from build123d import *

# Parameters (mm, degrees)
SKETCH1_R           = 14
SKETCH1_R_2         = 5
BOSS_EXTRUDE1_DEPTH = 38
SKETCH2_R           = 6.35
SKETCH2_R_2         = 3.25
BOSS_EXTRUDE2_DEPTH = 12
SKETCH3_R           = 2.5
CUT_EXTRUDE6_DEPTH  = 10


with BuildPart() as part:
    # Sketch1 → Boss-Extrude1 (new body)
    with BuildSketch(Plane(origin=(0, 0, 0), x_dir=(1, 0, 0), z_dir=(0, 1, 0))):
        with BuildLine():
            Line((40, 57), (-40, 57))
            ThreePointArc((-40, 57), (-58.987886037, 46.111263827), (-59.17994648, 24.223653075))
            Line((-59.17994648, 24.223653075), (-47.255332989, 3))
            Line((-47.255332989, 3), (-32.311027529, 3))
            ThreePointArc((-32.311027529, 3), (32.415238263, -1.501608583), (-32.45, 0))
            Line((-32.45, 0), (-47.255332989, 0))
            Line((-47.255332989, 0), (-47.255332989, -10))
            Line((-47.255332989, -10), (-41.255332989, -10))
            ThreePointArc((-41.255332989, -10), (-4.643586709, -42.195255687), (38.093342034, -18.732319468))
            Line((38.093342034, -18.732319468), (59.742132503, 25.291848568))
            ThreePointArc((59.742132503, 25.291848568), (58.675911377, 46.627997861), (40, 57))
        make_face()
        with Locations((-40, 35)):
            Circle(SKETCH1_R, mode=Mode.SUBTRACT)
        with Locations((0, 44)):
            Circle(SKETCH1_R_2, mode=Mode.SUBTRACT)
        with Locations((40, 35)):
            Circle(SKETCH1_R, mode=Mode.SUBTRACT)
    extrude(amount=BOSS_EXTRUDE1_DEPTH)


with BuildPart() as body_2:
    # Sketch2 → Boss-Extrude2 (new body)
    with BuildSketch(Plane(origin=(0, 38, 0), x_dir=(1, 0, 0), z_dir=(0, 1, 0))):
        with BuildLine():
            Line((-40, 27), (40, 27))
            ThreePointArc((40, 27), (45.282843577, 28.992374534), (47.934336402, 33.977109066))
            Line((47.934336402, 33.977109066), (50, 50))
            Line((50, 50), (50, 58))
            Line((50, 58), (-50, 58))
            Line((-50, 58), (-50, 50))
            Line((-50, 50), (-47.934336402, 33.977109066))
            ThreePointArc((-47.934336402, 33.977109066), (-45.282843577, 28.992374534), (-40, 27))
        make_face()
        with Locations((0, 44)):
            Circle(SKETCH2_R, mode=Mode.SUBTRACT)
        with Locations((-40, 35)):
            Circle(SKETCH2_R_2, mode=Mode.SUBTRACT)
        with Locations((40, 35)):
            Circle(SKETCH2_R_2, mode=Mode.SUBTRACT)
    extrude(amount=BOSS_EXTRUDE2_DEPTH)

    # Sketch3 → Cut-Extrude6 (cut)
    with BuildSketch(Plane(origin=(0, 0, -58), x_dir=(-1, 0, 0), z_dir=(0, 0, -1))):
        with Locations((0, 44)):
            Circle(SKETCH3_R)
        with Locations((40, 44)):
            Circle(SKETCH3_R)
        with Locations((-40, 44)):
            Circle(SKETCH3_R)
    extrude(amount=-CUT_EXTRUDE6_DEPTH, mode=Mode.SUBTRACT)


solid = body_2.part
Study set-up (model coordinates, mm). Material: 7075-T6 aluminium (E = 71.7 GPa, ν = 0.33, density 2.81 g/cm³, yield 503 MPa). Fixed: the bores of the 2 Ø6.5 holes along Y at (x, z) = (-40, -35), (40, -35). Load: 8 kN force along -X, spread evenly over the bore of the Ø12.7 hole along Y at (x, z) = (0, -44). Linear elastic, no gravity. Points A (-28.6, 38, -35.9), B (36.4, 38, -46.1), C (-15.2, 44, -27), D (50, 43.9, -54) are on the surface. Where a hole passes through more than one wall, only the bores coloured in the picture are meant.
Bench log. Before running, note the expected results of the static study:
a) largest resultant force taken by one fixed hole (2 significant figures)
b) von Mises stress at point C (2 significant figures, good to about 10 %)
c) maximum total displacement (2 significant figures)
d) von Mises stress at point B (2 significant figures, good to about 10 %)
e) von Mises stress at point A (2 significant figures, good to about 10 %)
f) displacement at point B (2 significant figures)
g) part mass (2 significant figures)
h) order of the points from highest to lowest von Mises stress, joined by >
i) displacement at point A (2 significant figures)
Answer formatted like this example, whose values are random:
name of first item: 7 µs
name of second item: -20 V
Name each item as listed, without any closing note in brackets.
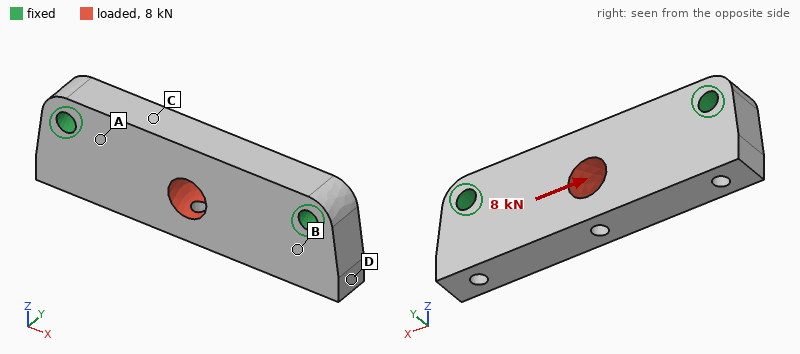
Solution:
largest resultant force taken by one fixed hole: 4.1 kN
von Mises stress at point C: 12 MPa
maximum total displacement: 10.0 µm
von Mises stress at point B: 7.3 MPa
von Mises stress at point A: 19 MPa
displacement at point B: 3.9 µm
part mass: 94 g
order of the points from highest to lowest von Mises stress, joined by >: A > C > B > D
displacement at point A: 2.8 µm
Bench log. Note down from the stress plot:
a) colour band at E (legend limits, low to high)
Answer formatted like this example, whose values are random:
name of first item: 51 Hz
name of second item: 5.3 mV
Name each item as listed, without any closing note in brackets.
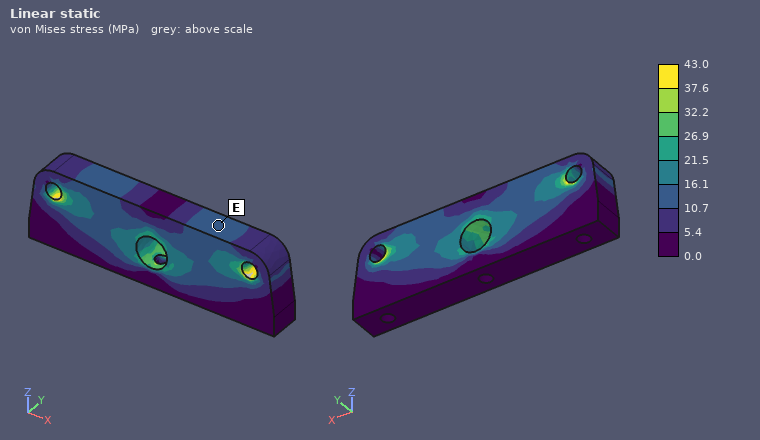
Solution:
colour band at E: 10.7 to 16.1 MPa
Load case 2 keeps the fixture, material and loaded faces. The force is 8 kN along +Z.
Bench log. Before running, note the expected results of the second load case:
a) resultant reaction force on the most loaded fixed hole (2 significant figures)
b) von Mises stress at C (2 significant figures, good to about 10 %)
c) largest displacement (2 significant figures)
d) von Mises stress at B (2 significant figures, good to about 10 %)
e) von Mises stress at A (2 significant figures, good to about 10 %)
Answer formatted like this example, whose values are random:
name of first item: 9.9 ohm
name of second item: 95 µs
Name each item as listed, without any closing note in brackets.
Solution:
resultant reaction force on the most loaded fixed hole: 4.7 kN
von Mises stress at C: 19 MPa
largest displacement: 43 µm
von Mises stress at B: 14 MPa
von Mises stress at A: 28 MPa
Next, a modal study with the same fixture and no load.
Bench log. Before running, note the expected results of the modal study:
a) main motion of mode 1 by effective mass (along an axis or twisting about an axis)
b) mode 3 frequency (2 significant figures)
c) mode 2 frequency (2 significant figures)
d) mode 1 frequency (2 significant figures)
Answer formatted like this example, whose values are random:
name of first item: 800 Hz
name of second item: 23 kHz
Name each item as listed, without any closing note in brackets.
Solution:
main motion of mode 1 by effective mass: along Y
mode 3 frequency: 12 kHz
mode 2 frequency: 11 kHz
mode 1 frequency: 7200 Hz
